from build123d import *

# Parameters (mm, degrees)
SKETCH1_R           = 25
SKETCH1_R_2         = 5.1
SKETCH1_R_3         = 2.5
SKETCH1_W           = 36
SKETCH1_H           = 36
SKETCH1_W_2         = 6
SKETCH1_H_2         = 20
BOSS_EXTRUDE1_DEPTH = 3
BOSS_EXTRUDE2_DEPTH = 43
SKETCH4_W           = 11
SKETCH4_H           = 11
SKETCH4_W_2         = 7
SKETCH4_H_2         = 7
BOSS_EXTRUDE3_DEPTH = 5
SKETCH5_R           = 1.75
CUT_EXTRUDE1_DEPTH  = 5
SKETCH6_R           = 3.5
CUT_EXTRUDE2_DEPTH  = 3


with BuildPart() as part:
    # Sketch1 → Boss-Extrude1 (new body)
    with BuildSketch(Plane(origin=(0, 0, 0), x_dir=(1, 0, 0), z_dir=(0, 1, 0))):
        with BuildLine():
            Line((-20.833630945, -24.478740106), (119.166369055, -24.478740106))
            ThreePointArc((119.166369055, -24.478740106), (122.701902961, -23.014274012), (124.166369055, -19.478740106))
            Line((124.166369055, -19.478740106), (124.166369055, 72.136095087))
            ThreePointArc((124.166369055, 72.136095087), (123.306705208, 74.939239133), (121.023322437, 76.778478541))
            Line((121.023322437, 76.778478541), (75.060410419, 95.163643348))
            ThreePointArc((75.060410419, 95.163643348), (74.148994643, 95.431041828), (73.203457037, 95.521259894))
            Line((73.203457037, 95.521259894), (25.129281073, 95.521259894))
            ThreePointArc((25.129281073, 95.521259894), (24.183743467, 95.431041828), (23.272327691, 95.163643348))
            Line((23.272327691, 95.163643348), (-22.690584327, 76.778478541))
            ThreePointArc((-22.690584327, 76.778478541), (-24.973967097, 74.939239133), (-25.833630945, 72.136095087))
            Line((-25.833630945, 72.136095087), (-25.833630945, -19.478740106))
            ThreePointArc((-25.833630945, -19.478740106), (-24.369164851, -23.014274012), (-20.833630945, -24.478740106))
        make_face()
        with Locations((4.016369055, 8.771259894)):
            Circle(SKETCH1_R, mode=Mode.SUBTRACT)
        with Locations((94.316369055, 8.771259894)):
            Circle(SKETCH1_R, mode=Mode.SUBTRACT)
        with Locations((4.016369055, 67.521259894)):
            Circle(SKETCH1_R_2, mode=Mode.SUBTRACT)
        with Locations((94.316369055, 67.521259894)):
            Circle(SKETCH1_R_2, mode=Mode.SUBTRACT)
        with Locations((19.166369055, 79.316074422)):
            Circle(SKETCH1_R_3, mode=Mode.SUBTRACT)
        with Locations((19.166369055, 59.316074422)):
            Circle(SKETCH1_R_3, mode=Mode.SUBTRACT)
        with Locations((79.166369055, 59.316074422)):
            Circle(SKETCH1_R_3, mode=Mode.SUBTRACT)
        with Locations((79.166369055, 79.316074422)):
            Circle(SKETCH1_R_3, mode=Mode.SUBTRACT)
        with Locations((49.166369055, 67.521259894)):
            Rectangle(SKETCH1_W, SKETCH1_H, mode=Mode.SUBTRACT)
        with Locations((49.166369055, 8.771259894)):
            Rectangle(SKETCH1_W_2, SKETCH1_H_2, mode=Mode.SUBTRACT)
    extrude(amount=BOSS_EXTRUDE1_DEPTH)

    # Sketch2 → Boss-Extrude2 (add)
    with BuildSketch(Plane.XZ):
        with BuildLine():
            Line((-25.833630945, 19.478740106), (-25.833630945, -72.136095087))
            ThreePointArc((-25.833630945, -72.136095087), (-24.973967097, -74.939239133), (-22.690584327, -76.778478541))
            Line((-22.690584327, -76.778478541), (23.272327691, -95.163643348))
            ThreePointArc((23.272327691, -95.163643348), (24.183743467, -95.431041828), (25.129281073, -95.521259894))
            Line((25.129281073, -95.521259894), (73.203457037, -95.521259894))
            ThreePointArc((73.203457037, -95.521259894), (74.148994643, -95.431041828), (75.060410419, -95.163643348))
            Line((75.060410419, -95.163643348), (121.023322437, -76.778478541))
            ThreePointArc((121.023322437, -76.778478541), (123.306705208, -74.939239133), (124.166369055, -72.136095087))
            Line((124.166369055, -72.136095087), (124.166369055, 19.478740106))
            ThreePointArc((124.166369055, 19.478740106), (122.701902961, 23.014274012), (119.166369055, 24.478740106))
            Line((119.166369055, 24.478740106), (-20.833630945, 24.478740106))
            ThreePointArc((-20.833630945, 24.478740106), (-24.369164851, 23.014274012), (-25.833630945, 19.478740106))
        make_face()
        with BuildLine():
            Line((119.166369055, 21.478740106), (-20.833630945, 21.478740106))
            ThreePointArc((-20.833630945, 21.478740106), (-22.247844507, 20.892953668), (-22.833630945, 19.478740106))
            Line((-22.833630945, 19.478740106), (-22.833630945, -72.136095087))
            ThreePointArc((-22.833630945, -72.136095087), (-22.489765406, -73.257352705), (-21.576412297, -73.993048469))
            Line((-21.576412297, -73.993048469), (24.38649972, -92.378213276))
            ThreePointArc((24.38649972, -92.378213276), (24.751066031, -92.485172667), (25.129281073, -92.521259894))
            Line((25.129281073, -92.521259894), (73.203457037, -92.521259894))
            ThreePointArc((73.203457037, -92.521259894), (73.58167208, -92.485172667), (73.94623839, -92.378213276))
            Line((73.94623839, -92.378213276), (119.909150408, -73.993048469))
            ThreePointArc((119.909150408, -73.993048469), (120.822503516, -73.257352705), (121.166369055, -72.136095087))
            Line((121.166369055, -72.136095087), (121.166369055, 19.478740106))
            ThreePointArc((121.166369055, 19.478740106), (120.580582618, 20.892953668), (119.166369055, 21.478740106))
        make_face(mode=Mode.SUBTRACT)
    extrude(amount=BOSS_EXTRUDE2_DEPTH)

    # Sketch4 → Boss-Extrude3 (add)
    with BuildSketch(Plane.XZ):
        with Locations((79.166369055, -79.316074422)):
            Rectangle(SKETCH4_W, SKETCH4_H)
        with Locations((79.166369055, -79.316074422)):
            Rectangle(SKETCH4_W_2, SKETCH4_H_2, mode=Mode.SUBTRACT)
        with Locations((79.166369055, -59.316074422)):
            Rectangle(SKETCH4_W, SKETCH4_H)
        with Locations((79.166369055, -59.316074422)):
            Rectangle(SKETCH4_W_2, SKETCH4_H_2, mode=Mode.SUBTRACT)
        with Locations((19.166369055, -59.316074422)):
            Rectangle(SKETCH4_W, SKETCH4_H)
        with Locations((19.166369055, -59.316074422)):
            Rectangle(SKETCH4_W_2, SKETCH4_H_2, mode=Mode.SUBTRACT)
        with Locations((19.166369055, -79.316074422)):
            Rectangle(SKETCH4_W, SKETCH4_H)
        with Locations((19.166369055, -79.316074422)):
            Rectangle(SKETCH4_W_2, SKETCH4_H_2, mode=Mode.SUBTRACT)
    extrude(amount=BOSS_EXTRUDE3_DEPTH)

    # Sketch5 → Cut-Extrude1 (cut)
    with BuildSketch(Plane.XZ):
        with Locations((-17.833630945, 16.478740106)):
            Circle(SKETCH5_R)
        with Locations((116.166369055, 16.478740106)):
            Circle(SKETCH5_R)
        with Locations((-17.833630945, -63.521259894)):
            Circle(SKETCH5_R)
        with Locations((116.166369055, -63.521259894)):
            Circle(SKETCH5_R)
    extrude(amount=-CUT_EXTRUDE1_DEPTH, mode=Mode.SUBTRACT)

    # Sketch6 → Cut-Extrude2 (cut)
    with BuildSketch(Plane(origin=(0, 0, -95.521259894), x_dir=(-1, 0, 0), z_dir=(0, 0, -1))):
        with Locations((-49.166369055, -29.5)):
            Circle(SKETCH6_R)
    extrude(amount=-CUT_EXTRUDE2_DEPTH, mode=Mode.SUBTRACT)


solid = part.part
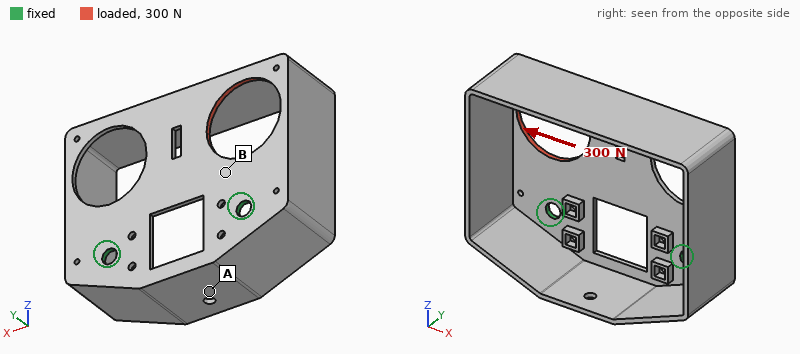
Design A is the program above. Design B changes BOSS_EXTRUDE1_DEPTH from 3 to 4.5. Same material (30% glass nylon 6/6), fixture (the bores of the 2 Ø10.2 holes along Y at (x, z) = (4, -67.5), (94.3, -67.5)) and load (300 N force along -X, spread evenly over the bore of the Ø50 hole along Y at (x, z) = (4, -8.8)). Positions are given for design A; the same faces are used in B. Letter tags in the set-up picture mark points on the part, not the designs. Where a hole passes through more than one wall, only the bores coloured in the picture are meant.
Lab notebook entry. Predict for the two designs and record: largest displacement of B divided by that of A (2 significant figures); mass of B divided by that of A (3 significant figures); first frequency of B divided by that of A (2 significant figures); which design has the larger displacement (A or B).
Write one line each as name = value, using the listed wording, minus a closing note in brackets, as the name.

largest displacement of B divided by that of A = 0.69
mass of B divided by that of A = 1.17
first frequency of B divided by that of A = 1.5
which design has the larger displacement = A
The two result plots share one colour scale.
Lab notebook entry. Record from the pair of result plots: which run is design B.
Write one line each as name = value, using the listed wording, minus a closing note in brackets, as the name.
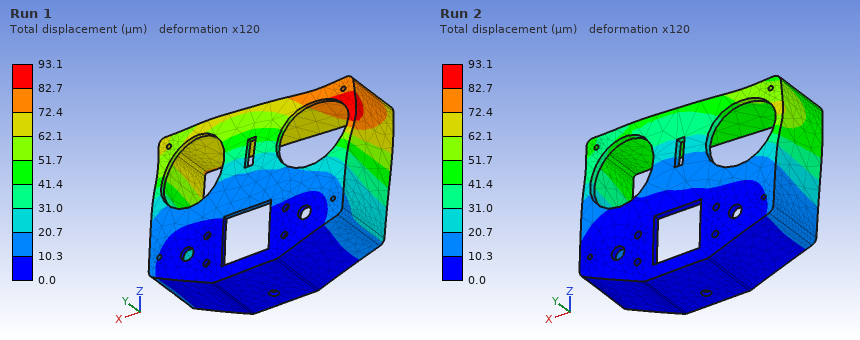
which run is design B = Run 2
